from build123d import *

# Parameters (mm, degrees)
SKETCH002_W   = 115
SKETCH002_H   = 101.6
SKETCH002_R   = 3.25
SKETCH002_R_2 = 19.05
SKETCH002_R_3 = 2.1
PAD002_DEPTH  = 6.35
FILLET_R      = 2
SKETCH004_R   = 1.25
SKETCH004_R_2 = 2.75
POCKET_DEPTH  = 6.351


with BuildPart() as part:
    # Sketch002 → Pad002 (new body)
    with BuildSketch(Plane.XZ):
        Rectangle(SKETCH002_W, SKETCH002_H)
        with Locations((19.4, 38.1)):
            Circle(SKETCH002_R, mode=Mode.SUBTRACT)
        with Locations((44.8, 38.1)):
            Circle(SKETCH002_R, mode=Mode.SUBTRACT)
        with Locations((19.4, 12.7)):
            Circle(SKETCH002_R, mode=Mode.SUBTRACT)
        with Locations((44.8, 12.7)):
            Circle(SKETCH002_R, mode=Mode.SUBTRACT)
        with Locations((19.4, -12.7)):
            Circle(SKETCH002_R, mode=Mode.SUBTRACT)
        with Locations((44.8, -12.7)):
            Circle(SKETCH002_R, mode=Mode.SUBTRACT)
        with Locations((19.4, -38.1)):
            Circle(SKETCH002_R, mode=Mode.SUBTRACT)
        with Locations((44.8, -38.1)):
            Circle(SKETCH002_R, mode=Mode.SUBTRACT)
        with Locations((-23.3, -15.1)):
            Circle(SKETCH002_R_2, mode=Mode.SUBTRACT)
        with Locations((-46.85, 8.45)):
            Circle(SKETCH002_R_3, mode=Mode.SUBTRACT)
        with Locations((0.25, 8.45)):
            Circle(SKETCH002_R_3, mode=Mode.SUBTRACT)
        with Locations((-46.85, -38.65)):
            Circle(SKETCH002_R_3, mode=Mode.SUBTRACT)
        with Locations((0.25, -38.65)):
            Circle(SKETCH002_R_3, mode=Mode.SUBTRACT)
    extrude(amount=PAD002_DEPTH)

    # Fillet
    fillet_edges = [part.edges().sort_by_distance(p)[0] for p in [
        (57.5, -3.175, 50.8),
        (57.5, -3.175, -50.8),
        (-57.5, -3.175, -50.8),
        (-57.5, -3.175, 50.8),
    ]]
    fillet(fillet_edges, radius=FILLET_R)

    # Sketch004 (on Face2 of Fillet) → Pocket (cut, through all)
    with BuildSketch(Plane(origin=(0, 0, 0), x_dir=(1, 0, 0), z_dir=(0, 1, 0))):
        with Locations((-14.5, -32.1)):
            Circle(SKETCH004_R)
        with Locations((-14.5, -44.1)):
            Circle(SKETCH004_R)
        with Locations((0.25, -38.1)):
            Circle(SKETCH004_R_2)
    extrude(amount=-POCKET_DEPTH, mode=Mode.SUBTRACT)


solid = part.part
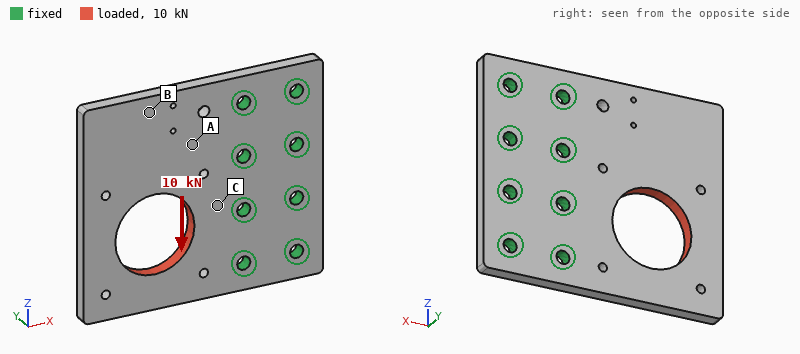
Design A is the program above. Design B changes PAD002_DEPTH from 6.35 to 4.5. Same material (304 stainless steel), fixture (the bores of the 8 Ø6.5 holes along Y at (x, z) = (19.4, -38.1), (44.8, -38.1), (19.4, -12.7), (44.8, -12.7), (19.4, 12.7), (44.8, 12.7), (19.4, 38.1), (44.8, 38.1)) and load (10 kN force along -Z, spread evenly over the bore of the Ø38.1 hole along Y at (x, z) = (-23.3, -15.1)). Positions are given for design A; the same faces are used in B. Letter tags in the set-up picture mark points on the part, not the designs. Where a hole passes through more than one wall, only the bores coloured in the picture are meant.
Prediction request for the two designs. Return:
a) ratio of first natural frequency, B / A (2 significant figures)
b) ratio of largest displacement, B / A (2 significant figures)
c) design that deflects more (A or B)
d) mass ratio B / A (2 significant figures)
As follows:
0.72
1.4
B
0.71
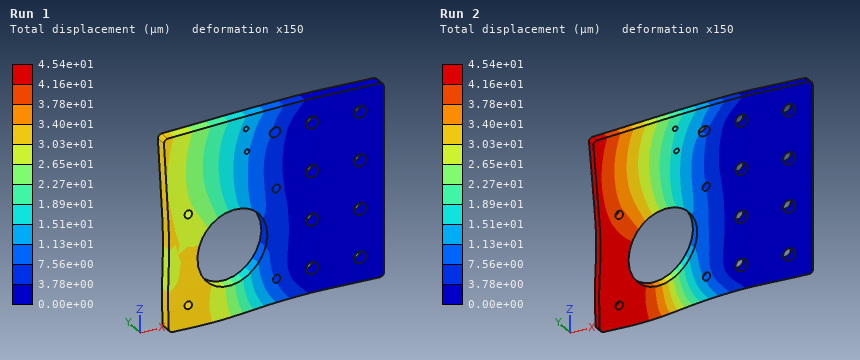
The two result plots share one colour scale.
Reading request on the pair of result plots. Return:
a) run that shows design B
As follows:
Run 2
